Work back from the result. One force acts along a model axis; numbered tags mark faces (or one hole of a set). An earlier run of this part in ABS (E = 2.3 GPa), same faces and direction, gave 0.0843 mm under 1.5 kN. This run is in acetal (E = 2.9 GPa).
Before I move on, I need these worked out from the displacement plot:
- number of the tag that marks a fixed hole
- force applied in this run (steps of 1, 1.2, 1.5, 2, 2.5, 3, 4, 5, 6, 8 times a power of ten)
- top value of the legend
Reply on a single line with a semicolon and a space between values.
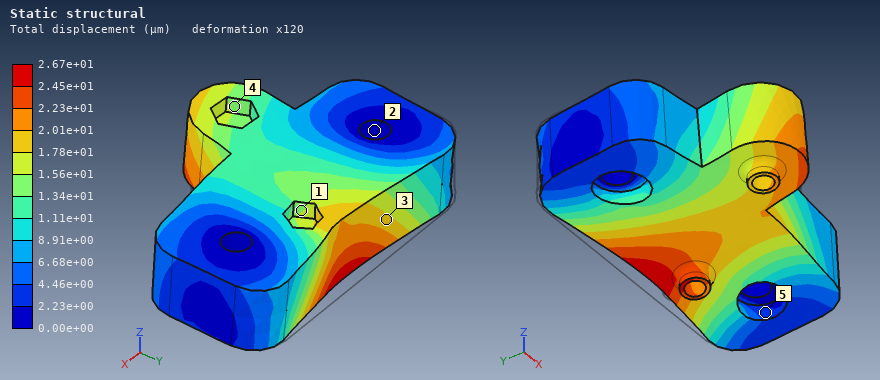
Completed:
2; 600 N; 2.67e+01 µm
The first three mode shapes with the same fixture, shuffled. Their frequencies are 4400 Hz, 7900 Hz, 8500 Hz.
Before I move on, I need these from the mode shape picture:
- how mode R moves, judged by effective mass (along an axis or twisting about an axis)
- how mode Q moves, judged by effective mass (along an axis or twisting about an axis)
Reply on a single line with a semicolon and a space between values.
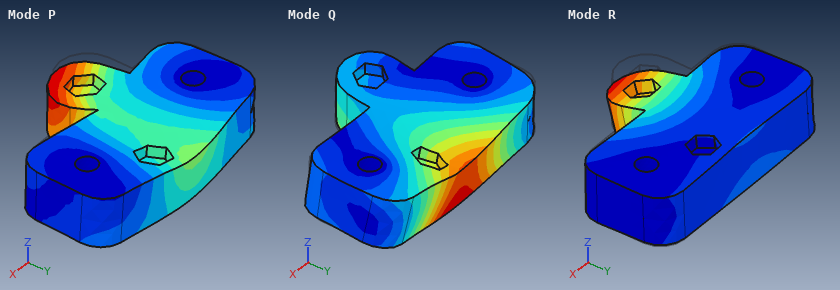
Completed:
along Z; along Z
